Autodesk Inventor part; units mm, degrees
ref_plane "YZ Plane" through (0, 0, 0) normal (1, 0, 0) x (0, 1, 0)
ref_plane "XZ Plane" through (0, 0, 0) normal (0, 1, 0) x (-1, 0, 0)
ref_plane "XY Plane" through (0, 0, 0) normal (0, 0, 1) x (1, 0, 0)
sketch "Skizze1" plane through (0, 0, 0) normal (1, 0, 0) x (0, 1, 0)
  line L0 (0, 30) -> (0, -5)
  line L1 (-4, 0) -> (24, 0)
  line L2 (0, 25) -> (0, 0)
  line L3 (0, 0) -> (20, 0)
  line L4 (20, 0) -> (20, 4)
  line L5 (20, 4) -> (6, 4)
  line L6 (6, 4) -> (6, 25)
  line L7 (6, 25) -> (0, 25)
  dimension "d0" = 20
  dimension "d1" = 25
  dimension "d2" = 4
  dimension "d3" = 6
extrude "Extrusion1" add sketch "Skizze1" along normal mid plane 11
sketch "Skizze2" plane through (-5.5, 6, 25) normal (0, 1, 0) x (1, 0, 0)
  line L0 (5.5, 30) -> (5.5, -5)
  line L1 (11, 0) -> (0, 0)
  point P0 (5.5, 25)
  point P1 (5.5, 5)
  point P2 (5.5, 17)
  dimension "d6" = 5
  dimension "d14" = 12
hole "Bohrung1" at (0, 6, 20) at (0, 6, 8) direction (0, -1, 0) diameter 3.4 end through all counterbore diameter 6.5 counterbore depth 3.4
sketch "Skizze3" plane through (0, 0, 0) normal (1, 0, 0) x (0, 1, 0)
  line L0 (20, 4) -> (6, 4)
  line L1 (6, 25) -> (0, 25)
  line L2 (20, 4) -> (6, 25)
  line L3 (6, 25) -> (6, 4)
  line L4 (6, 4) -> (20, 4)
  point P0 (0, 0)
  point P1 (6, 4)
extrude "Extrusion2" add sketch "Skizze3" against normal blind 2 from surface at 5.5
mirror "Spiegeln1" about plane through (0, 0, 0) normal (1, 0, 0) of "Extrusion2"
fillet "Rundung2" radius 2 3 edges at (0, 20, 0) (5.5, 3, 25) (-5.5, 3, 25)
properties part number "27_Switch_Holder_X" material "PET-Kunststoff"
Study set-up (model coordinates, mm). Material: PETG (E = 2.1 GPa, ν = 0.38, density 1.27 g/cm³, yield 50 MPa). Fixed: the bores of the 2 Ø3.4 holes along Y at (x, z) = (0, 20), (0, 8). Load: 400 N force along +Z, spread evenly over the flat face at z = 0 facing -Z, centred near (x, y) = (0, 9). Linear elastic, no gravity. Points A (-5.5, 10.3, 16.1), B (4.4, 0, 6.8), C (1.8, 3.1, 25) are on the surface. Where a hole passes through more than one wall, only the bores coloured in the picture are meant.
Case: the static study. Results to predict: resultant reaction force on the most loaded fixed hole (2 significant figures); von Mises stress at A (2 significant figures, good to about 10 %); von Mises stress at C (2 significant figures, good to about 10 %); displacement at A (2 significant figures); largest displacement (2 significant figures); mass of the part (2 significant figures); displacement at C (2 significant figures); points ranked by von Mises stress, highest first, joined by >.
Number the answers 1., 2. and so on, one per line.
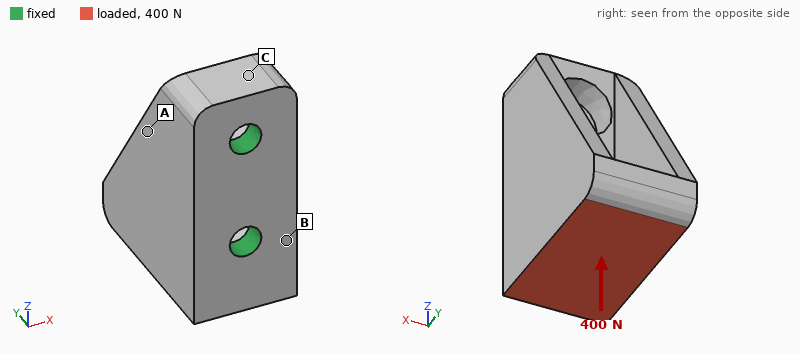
1. 310 N
2. 8.9 MPa
3. 2.9 MPa
4. 0.088 mm
5. 0.25 mm
6. 3.3 g
7. 0.043 mm
8. A > B > C
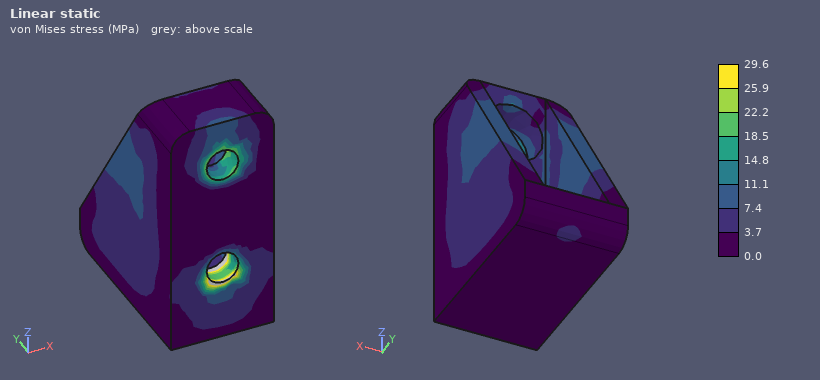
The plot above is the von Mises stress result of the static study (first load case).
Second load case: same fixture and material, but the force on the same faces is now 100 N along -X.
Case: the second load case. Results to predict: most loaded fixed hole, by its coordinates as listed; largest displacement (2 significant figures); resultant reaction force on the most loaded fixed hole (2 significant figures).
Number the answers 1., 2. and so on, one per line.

1. (0, 8)
2. 0.32 mm
3. 140 N
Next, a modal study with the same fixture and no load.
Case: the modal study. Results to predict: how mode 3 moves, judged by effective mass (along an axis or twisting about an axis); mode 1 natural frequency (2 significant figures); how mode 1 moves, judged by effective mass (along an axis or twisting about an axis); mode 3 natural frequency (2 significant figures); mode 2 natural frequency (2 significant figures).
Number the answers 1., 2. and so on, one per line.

1. twisting about Y
2. 2400 Hz
3. along X
4. 7600 Hz
5. 4800 Hz
